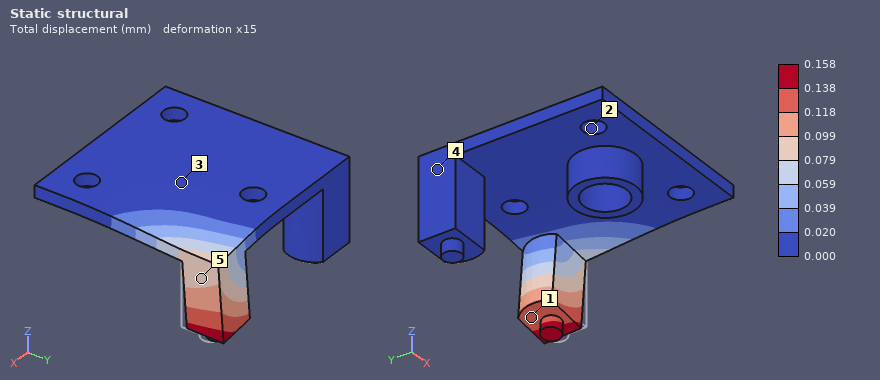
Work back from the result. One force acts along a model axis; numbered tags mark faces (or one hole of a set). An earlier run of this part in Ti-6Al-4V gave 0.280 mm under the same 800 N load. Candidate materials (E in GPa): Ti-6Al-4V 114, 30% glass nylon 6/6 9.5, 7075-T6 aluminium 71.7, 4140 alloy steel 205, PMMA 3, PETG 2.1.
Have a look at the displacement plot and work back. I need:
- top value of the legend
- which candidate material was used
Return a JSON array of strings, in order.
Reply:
["0.158 mm", "4140 alloy steel"]
